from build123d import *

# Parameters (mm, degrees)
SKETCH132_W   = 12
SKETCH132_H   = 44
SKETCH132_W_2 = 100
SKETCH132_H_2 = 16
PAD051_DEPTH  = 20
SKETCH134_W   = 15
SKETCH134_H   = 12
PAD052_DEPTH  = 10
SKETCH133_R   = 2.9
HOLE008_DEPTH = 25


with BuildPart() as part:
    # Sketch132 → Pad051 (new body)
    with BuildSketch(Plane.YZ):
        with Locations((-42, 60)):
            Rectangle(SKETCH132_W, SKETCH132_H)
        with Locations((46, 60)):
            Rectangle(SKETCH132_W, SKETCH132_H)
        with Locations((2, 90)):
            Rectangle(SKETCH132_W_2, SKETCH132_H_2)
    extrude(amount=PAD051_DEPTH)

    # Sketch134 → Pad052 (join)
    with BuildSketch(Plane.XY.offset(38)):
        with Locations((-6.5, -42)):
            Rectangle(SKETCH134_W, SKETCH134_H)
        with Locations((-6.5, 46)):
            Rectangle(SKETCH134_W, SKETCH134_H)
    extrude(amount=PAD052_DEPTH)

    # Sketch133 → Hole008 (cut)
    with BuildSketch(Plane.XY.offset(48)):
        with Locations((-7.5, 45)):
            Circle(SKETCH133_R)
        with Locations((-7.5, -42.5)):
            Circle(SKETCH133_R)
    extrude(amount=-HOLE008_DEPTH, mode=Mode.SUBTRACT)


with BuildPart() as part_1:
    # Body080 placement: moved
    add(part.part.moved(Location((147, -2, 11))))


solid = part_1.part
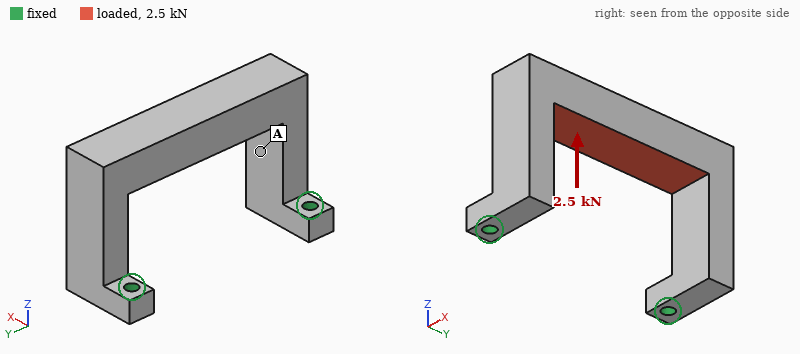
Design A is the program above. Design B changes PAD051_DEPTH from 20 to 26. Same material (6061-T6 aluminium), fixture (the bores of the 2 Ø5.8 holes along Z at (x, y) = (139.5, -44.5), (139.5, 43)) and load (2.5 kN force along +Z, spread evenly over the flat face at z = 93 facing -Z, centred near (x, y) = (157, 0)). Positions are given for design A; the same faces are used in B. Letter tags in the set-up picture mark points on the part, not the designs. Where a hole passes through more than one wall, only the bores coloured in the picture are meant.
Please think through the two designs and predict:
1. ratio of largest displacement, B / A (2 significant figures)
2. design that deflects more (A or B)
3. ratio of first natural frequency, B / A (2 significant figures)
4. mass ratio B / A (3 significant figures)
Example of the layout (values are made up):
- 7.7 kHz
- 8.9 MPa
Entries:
- 1.3
- B
- 0.88
- 1.28
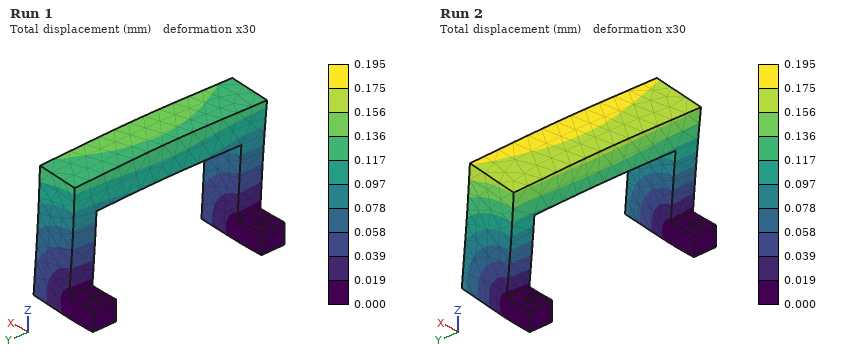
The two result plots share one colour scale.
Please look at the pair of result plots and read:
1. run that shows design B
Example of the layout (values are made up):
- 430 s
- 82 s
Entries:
- Run 2
